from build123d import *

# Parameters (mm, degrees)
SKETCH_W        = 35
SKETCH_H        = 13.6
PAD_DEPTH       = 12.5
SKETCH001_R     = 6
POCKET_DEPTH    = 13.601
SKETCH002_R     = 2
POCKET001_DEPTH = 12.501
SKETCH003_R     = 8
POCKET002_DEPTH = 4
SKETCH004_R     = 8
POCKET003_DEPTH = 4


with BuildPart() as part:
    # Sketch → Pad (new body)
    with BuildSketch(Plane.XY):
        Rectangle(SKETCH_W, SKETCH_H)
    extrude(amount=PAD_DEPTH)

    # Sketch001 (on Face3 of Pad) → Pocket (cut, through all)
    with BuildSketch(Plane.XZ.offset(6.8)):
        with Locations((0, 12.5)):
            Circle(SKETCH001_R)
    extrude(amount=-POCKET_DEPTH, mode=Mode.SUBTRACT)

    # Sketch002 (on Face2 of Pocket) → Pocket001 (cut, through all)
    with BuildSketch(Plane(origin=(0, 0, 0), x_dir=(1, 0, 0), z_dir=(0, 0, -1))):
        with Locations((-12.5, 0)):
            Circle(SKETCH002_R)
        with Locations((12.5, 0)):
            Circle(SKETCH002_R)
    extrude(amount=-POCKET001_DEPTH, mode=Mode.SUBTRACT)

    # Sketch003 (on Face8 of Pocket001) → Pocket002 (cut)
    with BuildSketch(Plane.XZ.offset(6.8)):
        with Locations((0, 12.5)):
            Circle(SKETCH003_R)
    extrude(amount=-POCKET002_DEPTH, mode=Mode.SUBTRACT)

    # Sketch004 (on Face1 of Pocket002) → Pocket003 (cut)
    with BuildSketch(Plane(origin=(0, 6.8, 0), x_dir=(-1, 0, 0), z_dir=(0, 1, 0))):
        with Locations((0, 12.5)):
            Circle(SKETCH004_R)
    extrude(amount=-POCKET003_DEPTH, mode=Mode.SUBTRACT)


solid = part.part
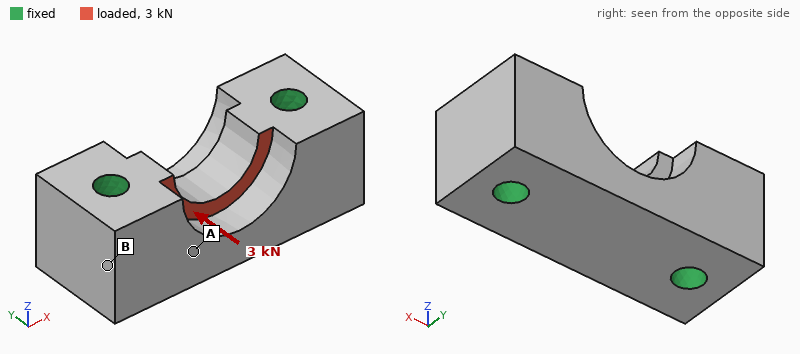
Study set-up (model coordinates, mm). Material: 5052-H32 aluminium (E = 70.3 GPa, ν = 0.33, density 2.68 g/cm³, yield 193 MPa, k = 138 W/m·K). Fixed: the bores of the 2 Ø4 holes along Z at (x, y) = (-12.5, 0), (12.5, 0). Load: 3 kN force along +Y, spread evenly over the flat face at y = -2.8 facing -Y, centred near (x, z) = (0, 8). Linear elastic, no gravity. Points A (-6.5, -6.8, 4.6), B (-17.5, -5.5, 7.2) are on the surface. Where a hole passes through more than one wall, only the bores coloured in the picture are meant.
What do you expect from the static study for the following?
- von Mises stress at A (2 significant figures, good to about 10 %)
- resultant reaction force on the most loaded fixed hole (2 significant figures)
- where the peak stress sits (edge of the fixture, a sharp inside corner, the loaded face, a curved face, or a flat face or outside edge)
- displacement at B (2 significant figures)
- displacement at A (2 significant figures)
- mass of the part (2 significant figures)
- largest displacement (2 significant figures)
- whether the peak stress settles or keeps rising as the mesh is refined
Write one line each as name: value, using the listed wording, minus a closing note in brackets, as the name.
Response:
von Mises stress at A: 16 MPa
resultant reaction force on the most loaded fixed hole: 1.5 kN
where the peak stress sits: edge of the fixture
displacement at B: 2.2 µm
displacement at A: 4.6 µm
mass of the part: 12 g
largest displacement: 10 µm
whether the peak stress settles or keeps rising as the mesh is refined: keeps rising
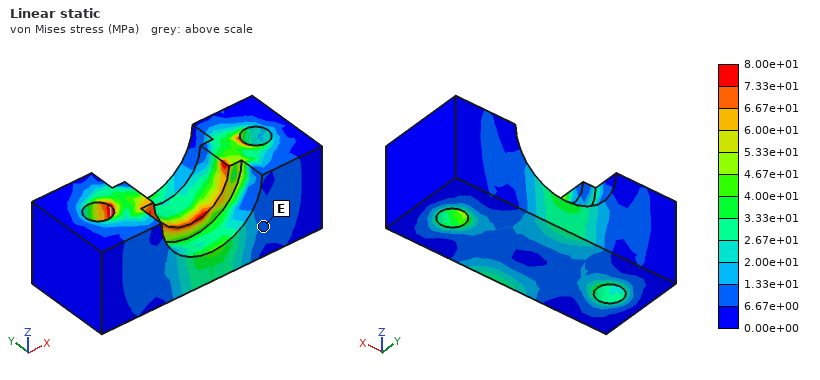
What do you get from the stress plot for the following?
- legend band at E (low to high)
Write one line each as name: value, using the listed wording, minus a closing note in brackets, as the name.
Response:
legend band at E: 6.67e+00 to 1.33e+01 MPa
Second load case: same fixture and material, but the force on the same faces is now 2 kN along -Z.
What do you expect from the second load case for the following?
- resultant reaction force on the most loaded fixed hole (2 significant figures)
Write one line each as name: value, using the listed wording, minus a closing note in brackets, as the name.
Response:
resultant reaction force on the most loaded fixed hole: 1.0 kN
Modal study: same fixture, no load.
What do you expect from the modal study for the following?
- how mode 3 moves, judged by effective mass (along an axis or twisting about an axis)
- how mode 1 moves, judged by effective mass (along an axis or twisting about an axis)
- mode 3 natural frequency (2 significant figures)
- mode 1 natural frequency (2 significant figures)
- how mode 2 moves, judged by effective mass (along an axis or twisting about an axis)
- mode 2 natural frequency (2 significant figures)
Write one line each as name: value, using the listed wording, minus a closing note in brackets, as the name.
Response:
how mode 3 moves, judged by effective mass: twisting about X
how mode 1 moves, judged by effective mass: along Y
mode 3 natural frequency: 75 kHz
mode 1 natural frequency: 49 kHz
how mode 2 moves, judged by effective mass: along Z
mode 2 natural frequency: 60 kHz
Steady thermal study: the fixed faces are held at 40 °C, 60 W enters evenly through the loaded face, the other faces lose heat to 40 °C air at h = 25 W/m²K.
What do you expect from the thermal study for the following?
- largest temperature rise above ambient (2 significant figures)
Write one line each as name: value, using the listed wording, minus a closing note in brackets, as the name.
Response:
largest temperature rise above ambient: 30 K
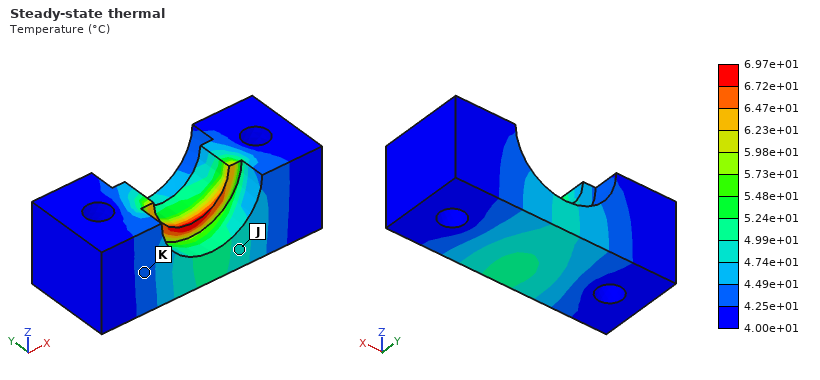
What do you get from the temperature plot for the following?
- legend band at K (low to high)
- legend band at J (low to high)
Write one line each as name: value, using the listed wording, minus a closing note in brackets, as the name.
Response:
legend band at K: 4.25e+01 to 4.49e+01 °C
legend band at J: 4.74e+01 to 4.99e+01 °C
